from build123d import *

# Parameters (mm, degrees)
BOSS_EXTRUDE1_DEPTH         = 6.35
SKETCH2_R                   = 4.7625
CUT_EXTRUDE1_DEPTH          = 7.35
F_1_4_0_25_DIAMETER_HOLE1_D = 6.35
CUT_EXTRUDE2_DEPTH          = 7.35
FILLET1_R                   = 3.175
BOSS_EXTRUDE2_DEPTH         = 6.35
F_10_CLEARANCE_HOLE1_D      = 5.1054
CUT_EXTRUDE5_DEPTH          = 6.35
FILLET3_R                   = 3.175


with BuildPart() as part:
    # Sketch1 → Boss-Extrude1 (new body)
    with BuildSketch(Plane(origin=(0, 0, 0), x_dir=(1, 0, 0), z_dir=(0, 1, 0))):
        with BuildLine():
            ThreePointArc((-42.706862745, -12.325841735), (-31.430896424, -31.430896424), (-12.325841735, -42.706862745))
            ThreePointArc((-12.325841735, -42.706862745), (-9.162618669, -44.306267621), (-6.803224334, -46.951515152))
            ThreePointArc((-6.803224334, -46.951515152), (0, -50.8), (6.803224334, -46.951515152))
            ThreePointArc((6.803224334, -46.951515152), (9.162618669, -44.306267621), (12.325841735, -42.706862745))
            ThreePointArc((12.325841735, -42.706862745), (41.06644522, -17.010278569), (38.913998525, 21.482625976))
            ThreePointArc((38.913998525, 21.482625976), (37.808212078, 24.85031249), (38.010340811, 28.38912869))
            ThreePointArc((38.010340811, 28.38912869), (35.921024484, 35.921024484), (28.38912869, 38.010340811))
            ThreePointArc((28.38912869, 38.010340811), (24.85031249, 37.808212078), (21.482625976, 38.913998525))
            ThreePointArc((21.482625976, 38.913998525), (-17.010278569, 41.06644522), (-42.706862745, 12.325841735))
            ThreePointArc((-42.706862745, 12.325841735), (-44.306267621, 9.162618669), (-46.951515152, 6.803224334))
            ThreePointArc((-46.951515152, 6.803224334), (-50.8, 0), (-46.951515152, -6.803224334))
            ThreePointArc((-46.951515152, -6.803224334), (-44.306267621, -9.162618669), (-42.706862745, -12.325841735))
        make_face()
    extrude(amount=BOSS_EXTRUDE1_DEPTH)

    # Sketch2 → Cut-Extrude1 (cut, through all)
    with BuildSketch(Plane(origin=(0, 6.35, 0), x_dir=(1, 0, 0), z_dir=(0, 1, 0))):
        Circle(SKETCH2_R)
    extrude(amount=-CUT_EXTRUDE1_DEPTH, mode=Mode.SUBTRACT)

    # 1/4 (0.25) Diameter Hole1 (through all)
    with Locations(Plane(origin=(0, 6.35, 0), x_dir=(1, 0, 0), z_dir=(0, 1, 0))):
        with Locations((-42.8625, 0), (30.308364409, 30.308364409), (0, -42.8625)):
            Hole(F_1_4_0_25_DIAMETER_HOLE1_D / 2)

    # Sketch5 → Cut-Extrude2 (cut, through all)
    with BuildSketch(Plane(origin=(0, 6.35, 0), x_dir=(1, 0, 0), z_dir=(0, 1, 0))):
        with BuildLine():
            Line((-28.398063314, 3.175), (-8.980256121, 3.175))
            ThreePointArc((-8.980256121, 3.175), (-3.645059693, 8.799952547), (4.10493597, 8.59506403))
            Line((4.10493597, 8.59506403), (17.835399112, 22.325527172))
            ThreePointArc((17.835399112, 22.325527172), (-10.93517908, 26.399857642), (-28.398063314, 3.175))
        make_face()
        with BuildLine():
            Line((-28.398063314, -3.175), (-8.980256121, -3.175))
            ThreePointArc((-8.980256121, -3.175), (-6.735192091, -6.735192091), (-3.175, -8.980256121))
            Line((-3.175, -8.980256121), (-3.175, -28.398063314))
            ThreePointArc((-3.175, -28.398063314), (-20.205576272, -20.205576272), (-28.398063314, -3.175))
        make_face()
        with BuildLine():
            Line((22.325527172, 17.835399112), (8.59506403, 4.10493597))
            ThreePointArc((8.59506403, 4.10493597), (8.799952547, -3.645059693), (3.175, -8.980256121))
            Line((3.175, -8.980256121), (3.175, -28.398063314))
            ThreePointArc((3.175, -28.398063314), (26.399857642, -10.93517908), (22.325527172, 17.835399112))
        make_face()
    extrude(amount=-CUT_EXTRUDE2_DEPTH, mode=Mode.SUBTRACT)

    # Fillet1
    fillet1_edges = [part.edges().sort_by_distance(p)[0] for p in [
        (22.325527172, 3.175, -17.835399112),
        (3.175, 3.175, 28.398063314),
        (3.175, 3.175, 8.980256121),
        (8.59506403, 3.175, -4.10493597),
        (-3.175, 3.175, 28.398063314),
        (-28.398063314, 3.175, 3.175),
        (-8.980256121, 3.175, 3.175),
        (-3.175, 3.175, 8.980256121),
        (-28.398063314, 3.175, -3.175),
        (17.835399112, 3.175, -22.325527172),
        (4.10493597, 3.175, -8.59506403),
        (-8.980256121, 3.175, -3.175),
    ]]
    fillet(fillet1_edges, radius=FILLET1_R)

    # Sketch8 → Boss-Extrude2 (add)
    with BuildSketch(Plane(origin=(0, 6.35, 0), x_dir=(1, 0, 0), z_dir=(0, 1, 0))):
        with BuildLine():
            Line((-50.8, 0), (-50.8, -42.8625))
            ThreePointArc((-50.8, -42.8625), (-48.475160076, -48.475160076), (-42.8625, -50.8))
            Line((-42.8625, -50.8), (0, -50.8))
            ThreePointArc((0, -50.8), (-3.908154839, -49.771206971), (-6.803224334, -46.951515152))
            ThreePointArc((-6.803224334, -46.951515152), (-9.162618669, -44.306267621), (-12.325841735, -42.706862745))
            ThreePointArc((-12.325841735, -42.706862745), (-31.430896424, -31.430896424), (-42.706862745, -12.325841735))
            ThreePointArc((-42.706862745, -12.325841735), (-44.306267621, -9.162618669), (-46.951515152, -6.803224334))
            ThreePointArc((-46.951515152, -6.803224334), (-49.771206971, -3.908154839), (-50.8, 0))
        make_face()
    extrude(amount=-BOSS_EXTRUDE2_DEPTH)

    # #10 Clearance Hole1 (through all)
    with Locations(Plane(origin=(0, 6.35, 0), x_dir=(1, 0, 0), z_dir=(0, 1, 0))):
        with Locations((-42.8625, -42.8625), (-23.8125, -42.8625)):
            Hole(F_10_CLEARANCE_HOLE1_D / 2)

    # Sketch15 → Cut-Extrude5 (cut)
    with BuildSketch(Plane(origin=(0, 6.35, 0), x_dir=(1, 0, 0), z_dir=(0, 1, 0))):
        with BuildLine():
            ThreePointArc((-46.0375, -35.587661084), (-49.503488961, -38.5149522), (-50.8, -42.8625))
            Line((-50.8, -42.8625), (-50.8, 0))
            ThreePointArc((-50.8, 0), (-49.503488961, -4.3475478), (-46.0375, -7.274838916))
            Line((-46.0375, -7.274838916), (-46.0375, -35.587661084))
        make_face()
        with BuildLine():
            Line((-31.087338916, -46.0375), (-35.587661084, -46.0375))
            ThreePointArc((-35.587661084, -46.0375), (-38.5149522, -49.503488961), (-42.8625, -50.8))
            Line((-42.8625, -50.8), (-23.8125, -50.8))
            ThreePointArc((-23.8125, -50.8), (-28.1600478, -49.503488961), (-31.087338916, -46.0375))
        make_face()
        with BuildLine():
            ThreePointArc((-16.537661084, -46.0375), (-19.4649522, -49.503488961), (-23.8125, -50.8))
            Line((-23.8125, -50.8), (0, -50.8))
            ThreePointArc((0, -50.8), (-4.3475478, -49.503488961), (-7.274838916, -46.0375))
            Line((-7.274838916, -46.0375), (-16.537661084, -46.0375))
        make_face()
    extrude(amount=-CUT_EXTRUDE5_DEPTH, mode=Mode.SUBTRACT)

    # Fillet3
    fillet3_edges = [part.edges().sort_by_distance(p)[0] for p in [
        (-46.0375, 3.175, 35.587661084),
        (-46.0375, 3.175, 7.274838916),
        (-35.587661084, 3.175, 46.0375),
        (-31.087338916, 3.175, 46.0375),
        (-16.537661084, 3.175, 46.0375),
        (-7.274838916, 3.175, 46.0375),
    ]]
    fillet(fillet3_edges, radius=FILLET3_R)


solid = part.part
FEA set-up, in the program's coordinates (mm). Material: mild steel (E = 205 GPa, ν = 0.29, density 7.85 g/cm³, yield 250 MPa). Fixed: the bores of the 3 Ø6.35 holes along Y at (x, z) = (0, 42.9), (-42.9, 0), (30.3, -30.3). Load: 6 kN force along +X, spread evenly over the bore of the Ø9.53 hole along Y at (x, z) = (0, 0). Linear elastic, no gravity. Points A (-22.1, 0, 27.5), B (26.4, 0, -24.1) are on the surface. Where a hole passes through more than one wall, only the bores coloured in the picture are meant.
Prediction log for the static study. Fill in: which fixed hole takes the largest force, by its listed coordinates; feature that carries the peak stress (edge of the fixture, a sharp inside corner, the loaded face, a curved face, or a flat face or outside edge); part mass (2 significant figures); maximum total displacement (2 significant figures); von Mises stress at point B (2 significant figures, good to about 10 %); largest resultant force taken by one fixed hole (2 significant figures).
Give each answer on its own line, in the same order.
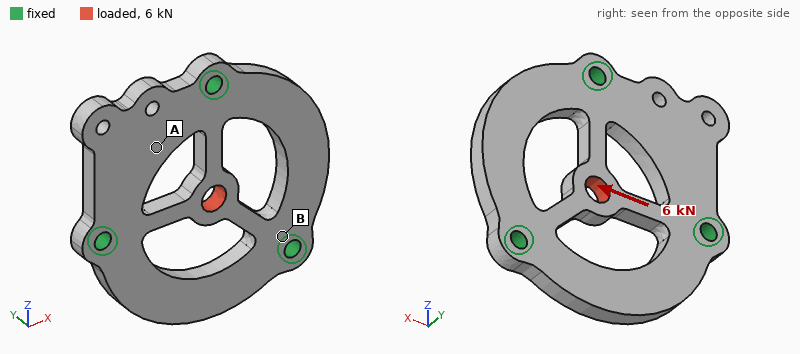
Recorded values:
(-42.9, 0)
a curved face
250 g
27 µm
34 MPa
3.8 kN
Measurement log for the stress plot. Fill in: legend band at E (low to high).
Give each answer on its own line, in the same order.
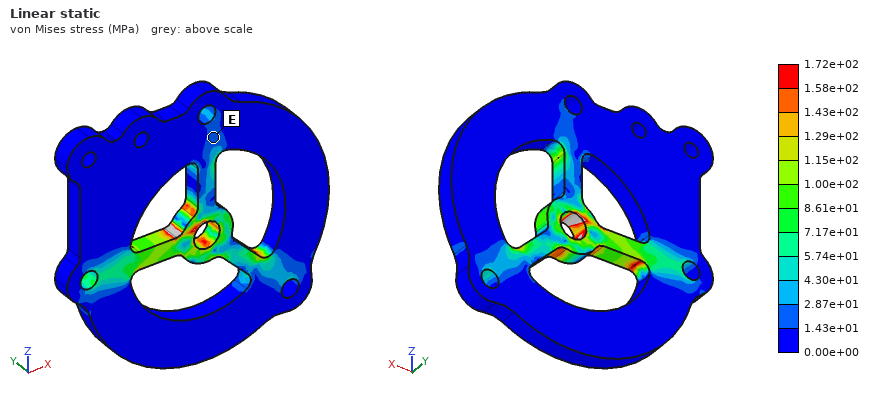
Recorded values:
1.43e+01 to 2.87e+01 MPa
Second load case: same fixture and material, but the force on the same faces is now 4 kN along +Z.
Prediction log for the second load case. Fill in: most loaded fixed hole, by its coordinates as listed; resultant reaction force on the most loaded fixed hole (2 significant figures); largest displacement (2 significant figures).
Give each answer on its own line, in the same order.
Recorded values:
(0, 42.9)
2.5 kN
18 µm
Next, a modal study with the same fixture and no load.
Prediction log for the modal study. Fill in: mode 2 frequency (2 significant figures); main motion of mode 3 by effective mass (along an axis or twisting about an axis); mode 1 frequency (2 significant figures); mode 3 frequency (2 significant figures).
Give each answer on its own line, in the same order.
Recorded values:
3800 Hz
along Y
3700 Hz
4000 Hz
